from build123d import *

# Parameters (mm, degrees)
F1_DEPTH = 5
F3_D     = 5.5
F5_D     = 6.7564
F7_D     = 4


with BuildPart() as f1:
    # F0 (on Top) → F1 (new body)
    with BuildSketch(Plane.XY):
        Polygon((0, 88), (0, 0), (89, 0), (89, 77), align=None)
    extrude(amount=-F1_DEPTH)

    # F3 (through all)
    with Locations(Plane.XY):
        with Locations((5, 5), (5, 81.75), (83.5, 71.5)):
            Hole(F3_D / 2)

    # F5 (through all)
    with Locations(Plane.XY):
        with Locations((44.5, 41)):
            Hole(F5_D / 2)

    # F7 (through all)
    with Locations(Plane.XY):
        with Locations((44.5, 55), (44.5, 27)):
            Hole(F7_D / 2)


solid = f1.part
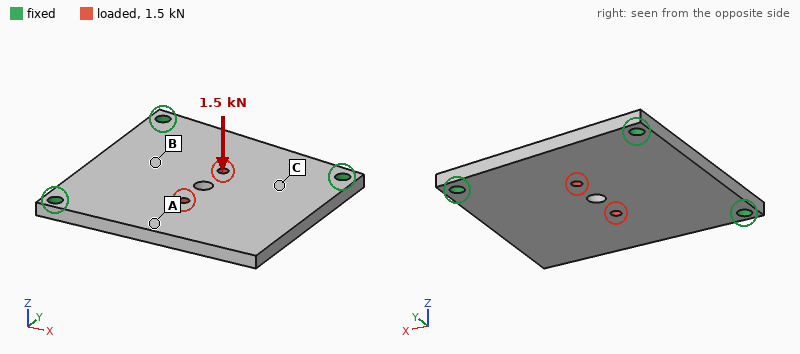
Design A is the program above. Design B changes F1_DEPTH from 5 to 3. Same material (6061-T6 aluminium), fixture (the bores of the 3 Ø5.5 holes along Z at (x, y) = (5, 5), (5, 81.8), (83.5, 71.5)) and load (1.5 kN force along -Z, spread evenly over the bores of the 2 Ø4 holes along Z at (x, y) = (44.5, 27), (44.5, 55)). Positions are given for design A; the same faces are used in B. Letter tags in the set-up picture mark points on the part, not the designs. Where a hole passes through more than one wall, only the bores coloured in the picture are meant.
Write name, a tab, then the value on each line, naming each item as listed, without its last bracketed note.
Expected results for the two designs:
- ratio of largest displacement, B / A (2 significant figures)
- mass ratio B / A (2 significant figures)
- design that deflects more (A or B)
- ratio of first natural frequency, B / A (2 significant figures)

ratio of largest displacement, B / A	4.3
mass ratio B / A	0.60
design that deflects more	B
ratio of first natural frequency, B / A	0.62
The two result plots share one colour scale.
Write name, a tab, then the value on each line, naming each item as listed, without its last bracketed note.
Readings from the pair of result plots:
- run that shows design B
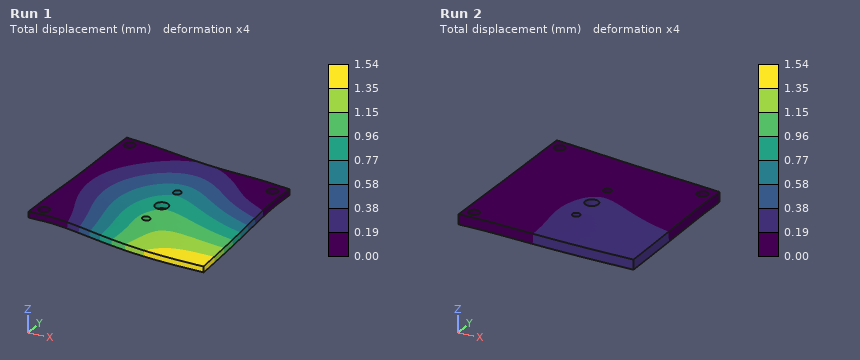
run that shows design B	Run 1
